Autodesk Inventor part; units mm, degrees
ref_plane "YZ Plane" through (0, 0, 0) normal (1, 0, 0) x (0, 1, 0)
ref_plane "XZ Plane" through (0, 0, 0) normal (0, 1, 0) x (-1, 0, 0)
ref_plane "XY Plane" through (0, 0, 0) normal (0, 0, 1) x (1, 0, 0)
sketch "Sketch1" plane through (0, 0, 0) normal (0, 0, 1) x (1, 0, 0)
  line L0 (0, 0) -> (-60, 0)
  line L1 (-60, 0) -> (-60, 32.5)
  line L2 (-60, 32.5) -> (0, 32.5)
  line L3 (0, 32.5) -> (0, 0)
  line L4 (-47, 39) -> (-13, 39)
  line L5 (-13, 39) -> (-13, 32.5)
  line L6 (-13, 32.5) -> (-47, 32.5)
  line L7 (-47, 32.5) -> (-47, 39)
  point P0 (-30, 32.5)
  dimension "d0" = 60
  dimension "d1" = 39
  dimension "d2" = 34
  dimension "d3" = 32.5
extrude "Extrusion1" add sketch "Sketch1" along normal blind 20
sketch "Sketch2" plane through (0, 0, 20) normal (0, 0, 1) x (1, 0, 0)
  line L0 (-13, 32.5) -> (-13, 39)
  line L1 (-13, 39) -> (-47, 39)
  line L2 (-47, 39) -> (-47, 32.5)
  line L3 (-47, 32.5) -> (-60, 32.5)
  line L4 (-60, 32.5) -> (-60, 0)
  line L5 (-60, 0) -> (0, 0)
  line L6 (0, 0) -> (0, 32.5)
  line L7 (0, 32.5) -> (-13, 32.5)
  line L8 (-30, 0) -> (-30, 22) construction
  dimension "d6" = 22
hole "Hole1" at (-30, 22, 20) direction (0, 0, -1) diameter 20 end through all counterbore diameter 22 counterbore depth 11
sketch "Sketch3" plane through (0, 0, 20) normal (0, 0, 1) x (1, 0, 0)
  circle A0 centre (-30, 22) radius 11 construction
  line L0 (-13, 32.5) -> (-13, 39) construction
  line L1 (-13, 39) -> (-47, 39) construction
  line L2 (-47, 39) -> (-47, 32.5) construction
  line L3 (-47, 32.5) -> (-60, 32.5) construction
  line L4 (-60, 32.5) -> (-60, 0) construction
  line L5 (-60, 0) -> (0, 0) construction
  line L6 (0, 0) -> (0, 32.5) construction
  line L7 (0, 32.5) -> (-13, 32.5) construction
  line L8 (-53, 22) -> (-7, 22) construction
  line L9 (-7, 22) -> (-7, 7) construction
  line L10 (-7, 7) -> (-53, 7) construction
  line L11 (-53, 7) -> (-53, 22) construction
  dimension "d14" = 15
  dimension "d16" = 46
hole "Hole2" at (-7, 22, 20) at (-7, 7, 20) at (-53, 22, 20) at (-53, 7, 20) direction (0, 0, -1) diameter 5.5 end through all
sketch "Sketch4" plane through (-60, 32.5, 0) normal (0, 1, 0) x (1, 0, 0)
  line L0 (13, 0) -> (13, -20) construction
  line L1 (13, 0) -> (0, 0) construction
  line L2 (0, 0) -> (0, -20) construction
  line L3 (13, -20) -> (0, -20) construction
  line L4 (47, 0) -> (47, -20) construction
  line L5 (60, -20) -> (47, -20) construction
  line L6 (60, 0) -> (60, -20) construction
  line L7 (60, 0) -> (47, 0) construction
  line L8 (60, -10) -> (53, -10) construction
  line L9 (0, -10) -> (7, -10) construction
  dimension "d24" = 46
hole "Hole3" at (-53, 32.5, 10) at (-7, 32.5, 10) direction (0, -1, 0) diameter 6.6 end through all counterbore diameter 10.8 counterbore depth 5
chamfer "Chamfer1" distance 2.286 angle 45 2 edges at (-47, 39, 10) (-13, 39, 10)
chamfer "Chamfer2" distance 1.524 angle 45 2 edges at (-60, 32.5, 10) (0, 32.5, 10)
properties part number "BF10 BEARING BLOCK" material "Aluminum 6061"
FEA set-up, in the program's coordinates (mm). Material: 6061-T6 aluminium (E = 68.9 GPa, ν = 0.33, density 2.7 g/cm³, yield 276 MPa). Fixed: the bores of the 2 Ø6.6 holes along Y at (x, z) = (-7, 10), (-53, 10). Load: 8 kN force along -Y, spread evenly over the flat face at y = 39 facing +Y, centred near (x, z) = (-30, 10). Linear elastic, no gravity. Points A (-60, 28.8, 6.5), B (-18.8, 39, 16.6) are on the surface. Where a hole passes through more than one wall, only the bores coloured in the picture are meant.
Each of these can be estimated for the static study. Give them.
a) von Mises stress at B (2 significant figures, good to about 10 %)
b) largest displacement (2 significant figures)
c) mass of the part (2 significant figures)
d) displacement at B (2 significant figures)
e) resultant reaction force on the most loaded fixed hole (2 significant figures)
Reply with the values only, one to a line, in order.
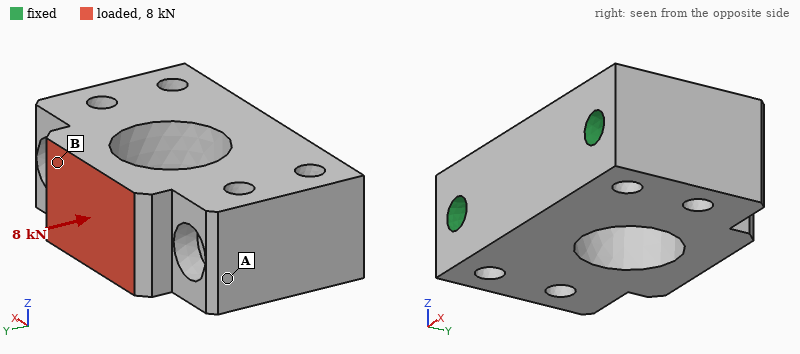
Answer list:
13 MPa
17 µm
87 g
9.6 µm
4.6 kN
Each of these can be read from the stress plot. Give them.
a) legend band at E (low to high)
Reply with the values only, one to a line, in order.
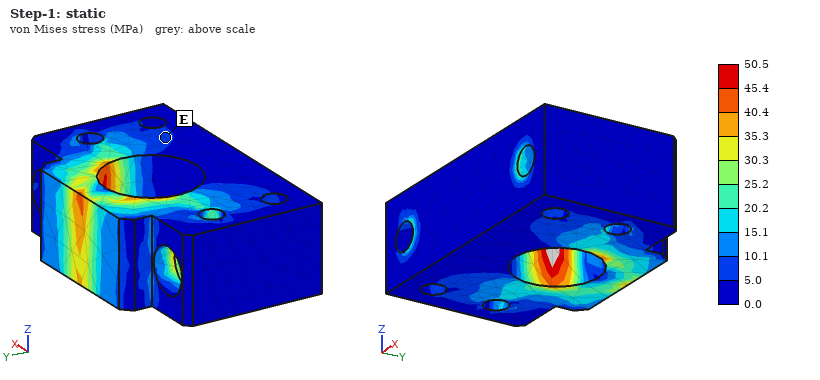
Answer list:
5.0 to 10.1 MPa
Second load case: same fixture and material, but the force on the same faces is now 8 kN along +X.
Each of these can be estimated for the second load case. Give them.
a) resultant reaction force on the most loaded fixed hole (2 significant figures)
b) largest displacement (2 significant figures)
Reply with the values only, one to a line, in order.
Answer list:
4.8 kN
18 µm
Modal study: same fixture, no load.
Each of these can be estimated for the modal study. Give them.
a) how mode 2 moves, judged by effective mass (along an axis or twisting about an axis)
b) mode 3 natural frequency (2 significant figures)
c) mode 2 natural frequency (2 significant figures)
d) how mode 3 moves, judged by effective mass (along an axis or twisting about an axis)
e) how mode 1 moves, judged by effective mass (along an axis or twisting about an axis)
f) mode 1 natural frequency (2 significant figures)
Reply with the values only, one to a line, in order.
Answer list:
along Z
29 kHz
25 kHz
along X
along Z
17 kHz
